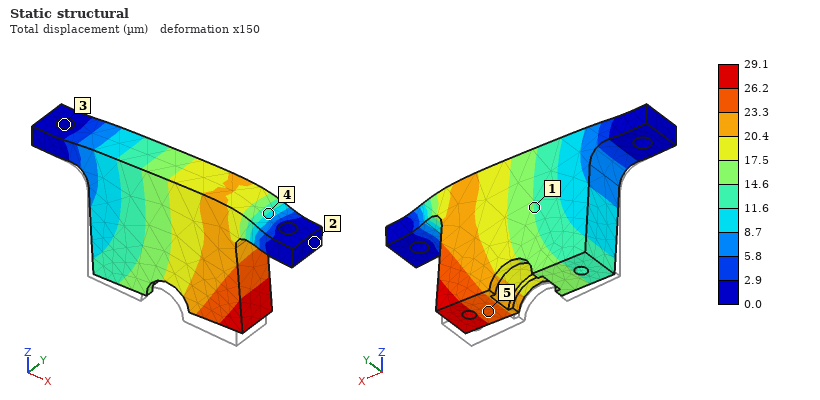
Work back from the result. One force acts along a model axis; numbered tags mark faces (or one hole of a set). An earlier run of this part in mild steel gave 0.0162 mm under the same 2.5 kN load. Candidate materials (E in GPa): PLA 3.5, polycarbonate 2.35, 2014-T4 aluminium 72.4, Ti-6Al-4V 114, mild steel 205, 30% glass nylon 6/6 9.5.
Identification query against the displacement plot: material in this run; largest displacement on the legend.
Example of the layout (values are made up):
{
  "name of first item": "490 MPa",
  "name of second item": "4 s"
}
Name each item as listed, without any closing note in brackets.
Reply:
{
  "material in this run": "Ti-6Al-4V",
  "largest displacement on the legend": "29.1 µm"
}
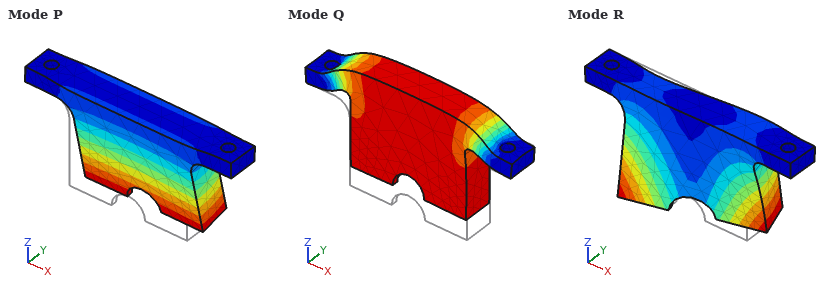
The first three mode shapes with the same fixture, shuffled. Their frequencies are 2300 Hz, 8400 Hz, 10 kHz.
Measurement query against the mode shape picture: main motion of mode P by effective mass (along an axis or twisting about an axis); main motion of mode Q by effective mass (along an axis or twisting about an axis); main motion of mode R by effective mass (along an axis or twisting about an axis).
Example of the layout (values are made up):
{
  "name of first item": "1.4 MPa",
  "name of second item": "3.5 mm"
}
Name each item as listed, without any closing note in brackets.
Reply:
{
  "main motion of mode P by effective mass": "along Y",
  "main motion of mode Q by effective mass": "along Z",
  "main motion of mode R by effective mass": "twisting about Z"
}
